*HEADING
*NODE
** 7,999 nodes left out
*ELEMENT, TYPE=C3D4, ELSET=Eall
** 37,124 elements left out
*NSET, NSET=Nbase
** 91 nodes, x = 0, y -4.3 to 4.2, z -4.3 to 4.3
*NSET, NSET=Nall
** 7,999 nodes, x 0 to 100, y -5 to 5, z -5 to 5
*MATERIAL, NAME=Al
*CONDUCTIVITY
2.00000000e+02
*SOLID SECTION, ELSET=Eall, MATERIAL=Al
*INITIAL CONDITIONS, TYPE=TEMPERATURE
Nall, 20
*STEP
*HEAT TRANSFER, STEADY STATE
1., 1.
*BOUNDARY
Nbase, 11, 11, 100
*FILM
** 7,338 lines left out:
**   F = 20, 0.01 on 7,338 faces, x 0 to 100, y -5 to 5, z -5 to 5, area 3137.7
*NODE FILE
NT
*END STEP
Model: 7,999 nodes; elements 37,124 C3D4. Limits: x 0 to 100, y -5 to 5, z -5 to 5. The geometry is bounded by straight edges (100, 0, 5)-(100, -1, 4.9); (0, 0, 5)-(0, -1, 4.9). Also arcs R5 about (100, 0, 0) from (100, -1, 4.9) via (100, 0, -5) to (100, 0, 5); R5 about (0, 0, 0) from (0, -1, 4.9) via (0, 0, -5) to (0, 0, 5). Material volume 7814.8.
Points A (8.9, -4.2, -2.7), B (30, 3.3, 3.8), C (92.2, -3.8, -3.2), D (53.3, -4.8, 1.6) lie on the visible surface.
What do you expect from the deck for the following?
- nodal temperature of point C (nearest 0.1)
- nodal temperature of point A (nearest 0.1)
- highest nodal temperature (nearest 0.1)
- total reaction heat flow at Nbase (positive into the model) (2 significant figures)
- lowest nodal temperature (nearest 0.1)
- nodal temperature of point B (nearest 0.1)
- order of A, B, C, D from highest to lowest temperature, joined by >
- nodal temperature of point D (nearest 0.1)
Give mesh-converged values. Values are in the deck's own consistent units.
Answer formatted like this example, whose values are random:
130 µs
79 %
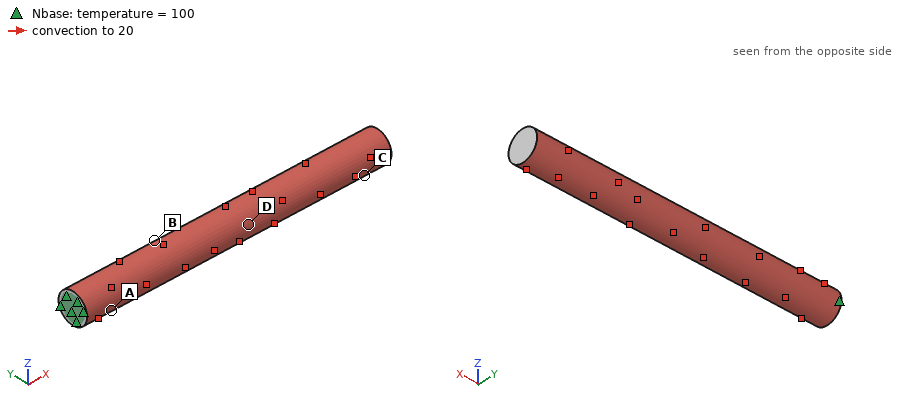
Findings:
92.6
98.7
100.0
2400
92.6
96.2
A > B > D > C
94.2
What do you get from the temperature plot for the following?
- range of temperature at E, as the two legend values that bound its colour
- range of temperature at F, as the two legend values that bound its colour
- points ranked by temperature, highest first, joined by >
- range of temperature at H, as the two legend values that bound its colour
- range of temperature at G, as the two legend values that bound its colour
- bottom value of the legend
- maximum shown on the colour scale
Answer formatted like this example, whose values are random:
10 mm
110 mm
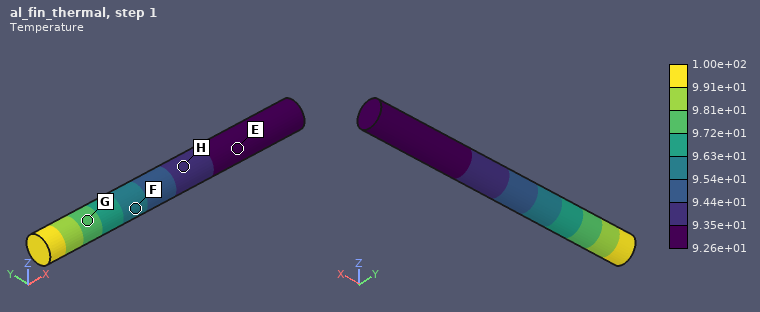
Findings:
9.26e+01 to 9.35e+01
9.54e+01 to 9.63e+01
G > F > H > E
9.35e+01 to 9.44e+01
9.72e+01 to 9.81e+01
9.26e+01
1.00e+02
